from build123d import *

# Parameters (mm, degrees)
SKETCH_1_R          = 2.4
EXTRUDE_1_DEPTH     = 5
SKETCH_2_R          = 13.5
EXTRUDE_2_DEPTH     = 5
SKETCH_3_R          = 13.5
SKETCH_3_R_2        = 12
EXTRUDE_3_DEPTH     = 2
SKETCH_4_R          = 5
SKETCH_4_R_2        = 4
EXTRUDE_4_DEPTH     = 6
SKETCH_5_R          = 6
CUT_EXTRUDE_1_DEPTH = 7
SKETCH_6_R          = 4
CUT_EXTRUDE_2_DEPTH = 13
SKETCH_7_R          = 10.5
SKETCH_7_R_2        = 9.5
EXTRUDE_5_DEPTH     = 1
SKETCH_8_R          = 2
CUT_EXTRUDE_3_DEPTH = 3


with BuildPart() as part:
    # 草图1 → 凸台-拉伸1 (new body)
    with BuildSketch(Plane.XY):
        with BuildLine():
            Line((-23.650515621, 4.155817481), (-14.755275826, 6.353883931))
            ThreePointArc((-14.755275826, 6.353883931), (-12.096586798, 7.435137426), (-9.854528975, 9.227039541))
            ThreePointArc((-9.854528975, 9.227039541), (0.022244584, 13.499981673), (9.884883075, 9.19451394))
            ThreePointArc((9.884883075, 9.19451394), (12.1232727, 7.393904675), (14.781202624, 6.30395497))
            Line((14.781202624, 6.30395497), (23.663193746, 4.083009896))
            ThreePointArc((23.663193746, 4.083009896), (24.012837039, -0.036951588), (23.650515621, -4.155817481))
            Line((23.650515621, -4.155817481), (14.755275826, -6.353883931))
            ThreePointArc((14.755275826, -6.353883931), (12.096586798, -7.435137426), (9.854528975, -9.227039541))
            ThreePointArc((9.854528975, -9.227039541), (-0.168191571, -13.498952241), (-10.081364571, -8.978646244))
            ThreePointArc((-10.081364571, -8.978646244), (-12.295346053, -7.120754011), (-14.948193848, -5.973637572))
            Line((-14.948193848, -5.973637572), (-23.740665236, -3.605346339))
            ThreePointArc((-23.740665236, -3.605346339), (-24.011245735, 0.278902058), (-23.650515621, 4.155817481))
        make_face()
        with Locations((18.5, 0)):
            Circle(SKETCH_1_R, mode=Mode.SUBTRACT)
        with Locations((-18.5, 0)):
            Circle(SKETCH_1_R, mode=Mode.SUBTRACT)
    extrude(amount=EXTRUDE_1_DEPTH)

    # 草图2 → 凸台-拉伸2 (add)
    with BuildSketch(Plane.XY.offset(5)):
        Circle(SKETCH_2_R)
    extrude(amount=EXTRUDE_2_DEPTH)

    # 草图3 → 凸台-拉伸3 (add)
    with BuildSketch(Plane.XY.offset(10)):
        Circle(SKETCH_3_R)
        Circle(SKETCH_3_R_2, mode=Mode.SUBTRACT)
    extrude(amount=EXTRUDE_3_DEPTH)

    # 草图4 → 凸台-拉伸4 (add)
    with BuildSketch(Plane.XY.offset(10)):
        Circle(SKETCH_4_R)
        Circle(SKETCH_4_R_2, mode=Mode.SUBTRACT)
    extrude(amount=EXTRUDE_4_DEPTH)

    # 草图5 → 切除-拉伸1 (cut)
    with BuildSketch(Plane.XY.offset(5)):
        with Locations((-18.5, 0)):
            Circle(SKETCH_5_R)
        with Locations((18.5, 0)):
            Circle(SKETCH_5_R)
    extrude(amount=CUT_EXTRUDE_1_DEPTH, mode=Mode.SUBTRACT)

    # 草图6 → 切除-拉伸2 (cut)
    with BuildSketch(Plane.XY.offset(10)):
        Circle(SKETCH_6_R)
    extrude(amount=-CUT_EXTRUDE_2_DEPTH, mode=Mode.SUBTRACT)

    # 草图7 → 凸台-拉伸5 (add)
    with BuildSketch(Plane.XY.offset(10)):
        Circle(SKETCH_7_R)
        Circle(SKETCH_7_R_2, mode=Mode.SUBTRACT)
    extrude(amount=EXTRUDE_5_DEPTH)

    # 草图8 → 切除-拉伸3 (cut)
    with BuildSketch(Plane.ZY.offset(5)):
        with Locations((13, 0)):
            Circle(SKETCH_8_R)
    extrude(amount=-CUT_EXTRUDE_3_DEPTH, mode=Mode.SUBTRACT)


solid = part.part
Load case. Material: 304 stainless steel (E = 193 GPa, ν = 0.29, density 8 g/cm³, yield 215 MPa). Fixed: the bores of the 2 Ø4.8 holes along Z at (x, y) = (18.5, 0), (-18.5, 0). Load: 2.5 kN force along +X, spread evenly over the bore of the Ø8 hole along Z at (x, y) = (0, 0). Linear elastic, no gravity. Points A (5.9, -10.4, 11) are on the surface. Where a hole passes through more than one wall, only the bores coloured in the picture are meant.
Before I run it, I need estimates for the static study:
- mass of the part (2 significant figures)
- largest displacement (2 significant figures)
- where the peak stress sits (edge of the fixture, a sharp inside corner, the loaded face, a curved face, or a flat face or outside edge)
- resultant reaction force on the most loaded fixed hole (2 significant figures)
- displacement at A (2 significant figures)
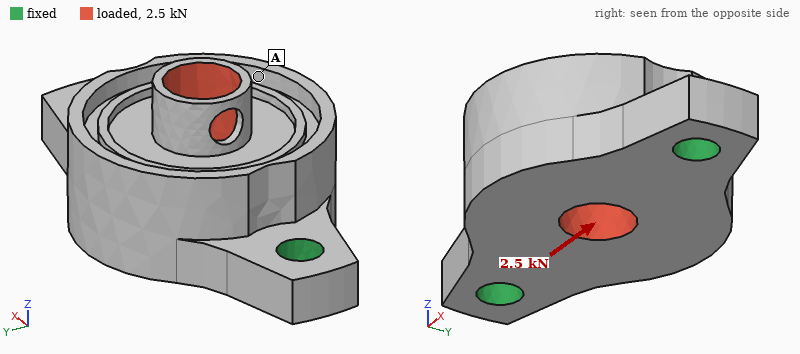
53 g
7.1 µm
the loaded face
1.3 kN
1.6 µm
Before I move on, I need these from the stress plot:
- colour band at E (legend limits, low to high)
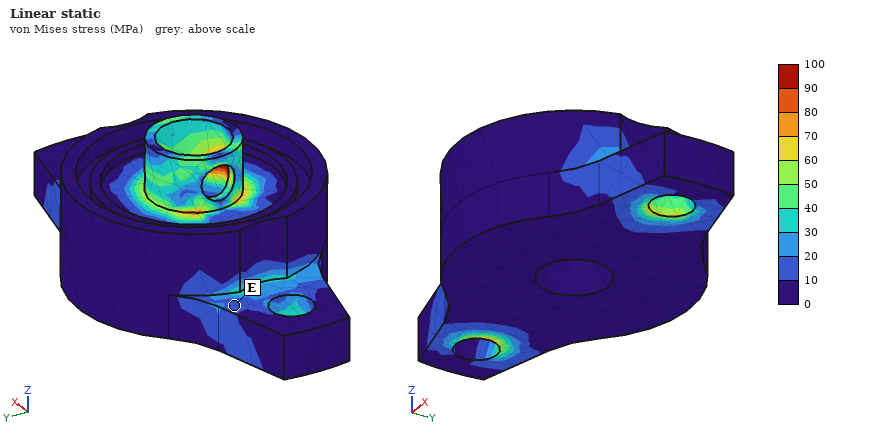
10 to 20 MPa
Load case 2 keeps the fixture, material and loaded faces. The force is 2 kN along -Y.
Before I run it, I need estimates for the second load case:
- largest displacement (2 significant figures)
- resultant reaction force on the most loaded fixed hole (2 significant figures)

22 µm
1.0 kN
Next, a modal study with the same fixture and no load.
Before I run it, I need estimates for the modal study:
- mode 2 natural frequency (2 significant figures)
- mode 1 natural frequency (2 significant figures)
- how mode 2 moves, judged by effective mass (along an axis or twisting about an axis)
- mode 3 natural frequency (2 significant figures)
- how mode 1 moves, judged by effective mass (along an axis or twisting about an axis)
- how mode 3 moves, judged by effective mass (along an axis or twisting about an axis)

16 kHz
9400 Hz
along Z
24 kHz
along Y
along Y
